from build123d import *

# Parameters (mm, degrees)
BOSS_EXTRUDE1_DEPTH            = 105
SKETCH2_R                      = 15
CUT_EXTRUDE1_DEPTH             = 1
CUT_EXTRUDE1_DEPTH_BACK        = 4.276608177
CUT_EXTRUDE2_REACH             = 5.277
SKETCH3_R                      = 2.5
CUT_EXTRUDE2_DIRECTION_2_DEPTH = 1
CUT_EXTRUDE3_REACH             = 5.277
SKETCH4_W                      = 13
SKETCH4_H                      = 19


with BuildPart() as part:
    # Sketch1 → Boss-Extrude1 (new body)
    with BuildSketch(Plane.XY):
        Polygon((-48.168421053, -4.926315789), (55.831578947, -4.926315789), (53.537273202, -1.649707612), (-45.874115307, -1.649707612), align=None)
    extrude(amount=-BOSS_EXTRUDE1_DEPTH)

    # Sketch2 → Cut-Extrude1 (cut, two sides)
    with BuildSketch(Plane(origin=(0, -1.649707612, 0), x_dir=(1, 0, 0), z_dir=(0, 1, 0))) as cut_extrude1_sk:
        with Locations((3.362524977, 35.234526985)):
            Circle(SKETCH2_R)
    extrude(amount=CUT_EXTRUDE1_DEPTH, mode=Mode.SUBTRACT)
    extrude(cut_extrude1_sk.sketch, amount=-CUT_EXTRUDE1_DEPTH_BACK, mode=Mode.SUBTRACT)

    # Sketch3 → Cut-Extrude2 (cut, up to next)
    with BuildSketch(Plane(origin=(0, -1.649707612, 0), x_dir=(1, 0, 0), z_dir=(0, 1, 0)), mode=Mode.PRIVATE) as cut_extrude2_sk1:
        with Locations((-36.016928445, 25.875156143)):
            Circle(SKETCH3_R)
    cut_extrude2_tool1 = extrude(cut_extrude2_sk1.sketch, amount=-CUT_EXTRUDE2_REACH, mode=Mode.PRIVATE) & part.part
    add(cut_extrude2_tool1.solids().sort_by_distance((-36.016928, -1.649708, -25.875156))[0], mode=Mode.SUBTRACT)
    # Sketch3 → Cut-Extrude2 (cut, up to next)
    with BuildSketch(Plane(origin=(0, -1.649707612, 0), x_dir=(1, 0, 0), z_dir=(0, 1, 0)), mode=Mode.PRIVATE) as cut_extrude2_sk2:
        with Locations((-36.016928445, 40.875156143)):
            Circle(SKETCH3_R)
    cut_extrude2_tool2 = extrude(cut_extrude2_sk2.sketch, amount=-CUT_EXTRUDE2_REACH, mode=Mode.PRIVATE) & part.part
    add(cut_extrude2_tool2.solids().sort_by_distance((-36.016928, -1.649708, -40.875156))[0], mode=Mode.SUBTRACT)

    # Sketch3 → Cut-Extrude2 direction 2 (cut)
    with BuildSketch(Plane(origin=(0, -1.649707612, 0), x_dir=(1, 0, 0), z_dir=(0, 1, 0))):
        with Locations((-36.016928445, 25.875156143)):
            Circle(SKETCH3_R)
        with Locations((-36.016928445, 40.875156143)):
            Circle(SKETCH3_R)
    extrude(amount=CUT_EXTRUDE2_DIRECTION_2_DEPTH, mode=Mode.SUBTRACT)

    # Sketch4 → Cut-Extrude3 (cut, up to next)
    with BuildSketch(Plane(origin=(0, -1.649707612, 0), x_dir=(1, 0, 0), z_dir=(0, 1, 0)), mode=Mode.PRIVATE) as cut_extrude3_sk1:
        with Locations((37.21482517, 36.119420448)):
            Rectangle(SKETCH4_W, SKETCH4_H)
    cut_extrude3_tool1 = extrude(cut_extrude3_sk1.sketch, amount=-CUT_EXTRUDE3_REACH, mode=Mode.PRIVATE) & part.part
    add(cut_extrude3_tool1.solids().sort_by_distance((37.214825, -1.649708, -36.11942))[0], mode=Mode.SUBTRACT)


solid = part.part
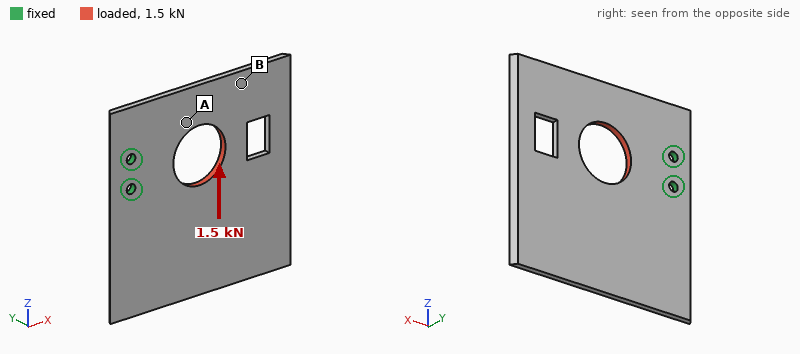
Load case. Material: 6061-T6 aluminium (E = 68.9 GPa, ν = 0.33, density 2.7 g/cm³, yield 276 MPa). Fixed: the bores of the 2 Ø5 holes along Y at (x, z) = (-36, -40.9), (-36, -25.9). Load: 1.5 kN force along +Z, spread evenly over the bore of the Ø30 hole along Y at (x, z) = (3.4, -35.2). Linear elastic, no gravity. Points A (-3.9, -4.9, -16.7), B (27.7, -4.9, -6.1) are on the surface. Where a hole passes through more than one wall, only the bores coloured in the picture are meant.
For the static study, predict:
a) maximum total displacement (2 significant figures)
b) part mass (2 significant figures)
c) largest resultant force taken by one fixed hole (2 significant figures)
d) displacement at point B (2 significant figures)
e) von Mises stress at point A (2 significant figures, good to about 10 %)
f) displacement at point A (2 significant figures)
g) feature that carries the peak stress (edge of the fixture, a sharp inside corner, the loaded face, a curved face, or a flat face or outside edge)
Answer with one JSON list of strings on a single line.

["0.20 mm", "86 g", "3.0 kN", "0.12 mm", "16 MPa", "0.060 mm", "edge of the fixture"]
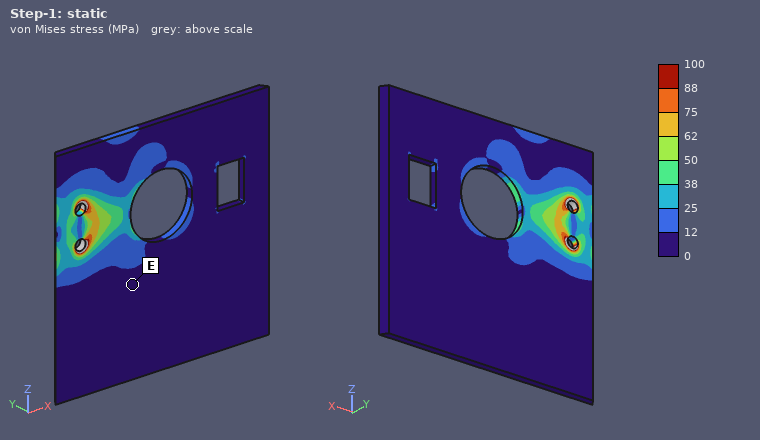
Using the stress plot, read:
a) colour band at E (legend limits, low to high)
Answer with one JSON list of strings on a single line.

["0 to 12 MPa"]
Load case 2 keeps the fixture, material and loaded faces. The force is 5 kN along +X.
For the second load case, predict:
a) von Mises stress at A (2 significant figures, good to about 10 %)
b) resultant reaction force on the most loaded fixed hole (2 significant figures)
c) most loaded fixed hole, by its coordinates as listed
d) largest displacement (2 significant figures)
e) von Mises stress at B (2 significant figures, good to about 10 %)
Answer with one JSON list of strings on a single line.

["34 MPa", "3.0 kN", "(-36, -40.9)", "47 µm", "9.1 MPa"]
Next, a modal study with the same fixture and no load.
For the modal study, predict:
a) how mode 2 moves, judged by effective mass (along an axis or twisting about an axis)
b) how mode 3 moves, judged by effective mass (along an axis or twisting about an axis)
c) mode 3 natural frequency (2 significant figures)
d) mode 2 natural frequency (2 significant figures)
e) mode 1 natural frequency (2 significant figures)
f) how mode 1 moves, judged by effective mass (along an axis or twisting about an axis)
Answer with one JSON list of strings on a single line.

["twisting about X", "along Y", "940 Hz", "440 Hz", "240 Hz", "along Y"]
